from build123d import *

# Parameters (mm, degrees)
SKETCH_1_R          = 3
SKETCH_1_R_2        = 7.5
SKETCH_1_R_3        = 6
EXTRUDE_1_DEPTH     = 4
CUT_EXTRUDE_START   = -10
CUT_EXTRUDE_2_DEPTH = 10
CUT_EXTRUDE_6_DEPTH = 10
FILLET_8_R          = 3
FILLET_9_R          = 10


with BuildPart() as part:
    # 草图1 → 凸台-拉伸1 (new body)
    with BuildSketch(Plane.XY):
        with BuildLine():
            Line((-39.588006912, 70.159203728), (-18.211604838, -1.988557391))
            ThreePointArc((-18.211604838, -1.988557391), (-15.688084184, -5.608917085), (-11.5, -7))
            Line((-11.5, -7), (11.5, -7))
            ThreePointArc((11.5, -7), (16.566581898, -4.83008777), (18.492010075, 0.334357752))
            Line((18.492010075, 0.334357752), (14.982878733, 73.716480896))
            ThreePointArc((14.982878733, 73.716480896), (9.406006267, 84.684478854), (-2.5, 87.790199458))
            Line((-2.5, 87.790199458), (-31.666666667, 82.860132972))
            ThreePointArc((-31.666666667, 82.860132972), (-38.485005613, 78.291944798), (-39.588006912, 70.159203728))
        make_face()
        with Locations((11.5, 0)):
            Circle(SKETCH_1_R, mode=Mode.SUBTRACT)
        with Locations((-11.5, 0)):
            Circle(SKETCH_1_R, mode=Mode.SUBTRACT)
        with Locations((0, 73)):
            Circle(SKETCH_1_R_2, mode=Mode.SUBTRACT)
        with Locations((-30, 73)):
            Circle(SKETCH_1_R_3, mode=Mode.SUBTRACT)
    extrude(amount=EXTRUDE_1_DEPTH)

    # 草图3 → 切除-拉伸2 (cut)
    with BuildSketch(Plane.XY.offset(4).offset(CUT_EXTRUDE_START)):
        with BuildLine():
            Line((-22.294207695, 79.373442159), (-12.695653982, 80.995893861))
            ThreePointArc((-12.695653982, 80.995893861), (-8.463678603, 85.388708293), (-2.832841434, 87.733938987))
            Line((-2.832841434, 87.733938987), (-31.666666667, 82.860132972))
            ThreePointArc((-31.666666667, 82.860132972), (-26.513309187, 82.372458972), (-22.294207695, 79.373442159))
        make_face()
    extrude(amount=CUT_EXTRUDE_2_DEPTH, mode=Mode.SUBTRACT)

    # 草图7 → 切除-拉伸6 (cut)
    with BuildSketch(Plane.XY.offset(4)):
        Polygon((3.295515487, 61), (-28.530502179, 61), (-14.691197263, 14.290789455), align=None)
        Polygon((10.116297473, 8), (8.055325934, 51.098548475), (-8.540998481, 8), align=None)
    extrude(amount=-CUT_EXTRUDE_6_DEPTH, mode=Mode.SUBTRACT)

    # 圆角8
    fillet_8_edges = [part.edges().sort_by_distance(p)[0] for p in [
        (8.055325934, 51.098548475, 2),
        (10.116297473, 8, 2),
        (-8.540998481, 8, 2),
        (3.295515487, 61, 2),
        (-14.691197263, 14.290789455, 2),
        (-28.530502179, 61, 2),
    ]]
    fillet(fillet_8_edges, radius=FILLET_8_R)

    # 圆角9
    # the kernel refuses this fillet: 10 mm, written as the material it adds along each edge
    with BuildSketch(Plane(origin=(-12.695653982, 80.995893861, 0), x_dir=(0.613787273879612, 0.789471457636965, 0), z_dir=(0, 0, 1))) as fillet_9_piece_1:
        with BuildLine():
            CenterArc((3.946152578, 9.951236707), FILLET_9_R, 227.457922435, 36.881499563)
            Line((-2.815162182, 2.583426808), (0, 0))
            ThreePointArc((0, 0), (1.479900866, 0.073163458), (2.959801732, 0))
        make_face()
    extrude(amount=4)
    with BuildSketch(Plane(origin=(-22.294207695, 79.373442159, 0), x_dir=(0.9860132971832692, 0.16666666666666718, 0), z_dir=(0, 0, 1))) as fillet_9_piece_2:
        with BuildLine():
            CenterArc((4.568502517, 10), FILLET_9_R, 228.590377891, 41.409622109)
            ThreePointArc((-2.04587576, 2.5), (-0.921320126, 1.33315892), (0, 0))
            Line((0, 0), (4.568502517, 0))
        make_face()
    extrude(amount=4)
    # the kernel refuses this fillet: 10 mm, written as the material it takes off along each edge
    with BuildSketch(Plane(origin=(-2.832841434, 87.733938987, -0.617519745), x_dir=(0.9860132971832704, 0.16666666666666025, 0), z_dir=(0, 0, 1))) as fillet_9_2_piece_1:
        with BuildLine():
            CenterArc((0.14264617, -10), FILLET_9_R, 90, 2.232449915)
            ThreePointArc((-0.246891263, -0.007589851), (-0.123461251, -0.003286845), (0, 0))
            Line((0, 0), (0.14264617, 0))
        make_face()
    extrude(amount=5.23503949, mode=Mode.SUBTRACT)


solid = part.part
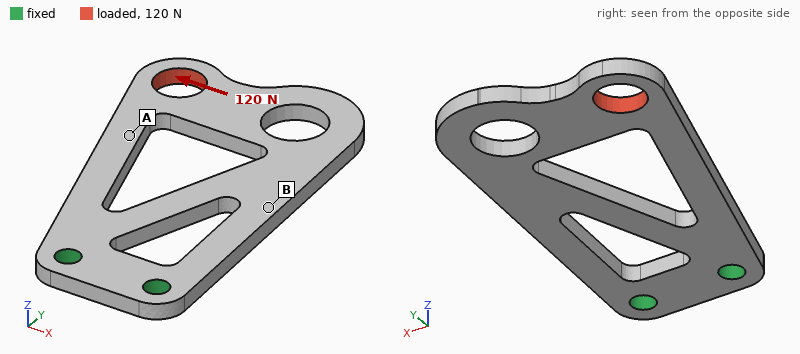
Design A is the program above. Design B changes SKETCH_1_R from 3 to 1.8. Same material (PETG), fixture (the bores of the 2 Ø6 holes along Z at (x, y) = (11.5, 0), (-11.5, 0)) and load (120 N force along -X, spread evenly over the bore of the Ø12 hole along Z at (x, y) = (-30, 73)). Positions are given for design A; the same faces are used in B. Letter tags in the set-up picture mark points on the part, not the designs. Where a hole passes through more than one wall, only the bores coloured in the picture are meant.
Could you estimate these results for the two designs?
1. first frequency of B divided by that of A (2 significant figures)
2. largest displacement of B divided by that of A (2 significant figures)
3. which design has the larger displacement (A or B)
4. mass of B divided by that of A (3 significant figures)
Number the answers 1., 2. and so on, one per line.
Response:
1. 0.97
2. 1.1
3. B
4. 1.01
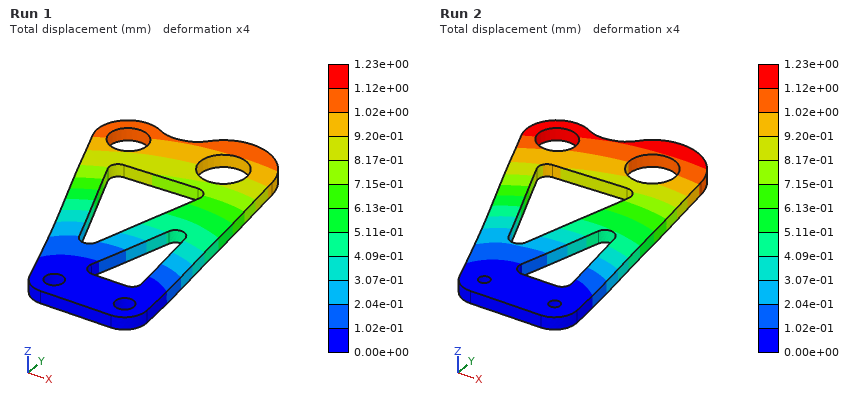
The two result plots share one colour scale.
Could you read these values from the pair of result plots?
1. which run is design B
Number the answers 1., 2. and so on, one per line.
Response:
1. Run 2
